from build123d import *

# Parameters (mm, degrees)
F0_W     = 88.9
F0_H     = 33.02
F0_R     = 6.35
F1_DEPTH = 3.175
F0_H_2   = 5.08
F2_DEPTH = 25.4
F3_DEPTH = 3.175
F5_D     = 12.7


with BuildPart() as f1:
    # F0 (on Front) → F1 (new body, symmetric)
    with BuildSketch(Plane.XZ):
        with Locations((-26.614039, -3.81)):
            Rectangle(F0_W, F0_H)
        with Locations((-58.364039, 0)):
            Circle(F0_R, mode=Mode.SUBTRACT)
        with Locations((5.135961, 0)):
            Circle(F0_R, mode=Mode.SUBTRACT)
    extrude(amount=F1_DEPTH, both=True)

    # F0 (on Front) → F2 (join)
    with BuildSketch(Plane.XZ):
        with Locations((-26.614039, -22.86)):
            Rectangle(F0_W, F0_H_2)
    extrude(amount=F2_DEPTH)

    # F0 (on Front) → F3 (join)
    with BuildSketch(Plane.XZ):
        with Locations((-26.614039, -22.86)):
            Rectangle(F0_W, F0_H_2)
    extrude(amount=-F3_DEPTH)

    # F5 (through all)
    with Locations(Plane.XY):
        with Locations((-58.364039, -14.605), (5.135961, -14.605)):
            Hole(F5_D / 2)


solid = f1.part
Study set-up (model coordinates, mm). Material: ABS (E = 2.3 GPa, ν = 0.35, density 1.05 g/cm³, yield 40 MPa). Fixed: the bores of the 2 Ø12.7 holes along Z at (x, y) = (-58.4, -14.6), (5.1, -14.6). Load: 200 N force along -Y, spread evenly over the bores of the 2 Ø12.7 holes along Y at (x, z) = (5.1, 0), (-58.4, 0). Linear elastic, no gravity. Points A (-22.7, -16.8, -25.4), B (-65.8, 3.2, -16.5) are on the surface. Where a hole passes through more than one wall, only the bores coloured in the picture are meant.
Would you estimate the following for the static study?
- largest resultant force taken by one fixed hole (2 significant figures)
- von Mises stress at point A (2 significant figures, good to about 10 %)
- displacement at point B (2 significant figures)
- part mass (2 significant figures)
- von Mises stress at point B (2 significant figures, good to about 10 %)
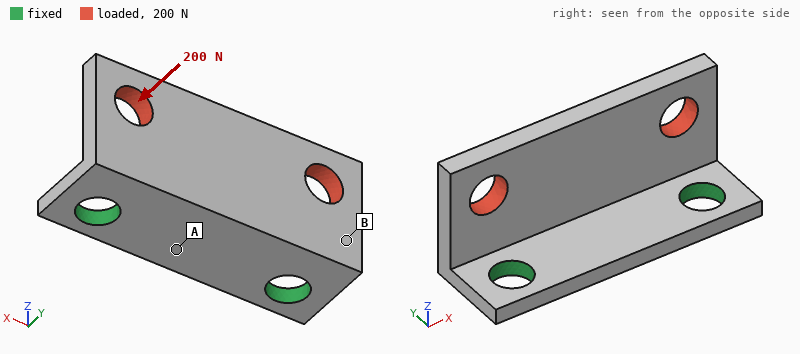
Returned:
100 N
2.8 MPa
0.26 mm
30 g
5.9 MPa
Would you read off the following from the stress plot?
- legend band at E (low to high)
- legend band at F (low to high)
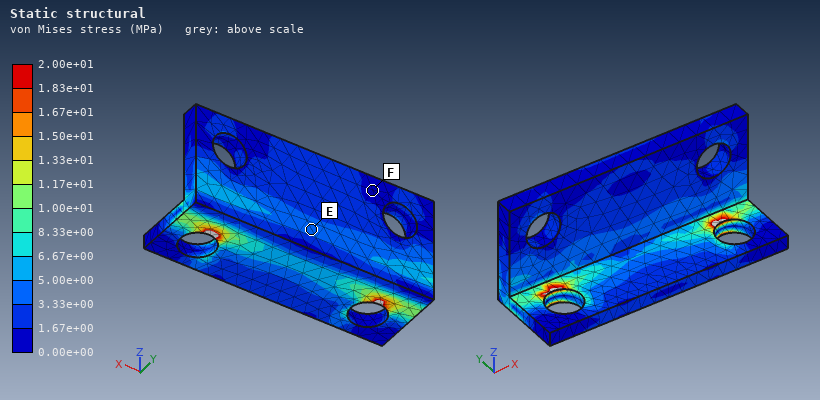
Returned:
3.33e+00 to 5.00e+00 MPa
0.00e+00 to 1.67e+00 MPa
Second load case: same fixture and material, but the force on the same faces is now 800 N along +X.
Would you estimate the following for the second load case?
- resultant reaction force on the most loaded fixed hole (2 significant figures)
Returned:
500 N
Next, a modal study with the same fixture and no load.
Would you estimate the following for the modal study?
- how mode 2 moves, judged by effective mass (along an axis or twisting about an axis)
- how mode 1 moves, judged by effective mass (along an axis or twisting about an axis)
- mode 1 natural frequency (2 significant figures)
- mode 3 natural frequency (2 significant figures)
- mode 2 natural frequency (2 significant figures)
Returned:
twisting about Z
along Y
680 Hz
2200 Hz
1200 Hz
